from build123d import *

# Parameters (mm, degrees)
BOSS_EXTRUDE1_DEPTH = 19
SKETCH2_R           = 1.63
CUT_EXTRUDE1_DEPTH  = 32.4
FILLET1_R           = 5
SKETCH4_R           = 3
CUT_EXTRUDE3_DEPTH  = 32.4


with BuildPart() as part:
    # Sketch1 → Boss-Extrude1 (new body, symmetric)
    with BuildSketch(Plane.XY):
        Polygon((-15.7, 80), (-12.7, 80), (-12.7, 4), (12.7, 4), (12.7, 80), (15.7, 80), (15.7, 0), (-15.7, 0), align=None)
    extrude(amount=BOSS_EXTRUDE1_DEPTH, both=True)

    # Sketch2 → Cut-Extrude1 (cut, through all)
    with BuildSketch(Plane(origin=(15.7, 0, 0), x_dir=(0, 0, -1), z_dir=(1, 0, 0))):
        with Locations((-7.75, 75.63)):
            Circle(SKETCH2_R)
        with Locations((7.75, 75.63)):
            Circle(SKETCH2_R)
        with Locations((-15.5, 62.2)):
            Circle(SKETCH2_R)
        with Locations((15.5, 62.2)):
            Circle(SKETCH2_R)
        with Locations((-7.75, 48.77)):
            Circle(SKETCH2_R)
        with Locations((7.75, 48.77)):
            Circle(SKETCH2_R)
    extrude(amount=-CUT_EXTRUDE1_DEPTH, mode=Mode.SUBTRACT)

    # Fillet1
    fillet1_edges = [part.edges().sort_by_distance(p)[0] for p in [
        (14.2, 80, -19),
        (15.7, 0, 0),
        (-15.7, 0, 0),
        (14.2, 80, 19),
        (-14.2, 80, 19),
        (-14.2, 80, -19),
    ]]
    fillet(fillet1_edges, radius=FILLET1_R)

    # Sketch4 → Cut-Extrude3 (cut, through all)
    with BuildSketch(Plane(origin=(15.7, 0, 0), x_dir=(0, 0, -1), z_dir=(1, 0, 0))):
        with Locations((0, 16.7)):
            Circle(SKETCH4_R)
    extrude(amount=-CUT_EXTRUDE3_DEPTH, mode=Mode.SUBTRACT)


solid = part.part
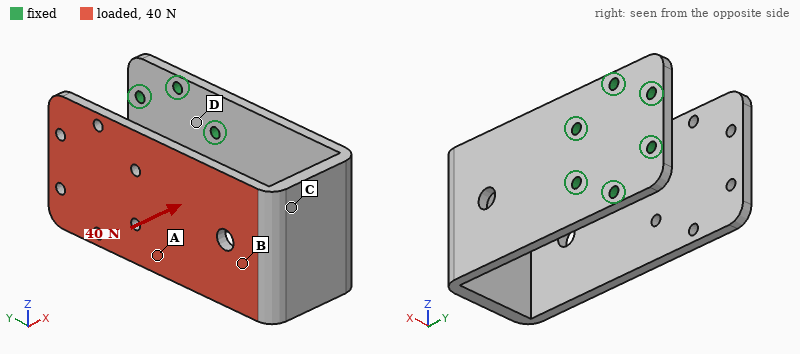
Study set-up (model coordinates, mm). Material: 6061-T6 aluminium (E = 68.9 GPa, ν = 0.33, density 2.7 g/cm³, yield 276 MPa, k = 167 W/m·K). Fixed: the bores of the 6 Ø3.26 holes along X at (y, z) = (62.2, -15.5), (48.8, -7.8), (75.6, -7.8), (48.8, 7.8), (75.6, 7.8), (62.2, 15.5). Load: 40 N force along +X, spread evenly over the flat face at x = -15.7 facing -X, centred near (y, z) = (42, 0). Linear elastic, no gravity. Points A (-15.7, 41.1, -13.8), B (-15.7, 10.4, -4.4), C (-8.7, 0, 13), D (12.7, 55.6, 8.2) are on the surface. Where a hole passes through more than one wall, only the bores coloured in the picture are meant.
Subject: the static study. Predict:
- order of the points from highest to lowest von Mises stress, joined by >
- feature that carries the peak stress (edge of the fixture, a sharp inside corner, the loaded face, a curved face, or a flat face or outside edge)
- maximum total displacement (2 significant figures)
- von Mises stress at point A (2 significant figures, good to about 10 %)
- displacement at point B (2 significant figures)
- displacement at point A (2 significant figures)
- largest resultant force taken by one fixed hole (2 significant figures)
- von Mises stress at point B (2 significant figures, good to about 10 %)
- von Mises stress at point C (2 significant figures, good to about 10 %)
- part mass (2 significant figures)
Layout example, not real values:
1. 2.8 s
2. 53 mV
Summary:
1. B > C > A > D
2. the loaded face
3. 1.0 mm
4. 7.1 MPa
5. 0.21 mm
6. 0.46 mm
7. 22 N
8. 20 MPa
9. 13 MPa
10. 57 g
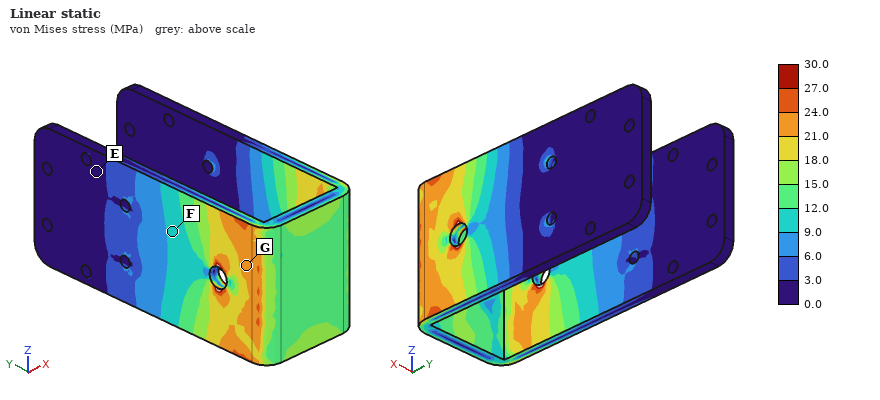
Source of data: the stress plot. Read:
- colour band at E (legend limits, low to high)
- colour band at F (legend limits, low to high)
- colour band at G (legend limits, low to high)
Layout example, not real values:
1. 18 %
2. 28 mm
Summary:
1. 0.0 to 3.0 MPa
2. 9.0 to 12.0 MPa
3. 21.0 to 24.0 MPa
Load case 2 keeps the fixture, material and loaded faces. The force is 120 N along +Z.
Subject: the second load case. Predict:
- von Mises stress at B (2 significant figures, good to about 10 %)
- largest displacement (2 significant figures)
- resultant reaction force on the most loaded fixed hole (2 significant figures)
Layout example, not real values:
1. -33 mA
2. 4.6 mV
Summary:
1. 9.5 MPa
2. 1.1 mm
3. 200 N
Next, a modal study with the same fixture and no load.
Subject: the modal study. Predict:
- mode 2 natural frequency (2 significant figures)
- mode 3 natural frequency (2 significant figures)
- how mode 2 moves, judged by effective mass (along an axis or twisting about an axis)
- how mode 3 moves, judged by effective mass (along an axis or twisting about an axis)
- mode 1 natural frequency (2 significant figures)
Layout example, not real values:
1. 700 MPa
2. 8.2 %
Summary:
1. 390 Hz
2. 430 Hz
3. along Z
4. along X
5. 220 Hz
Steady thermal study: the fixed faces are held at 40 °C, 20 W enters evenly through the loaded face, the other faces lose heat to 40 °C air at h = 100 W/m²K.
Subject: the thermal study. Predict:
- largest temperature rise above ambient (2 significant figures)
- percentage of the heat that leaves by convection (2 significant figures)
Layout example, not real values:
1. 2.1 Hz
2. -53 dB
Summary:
1. 35 K
2. 82 %
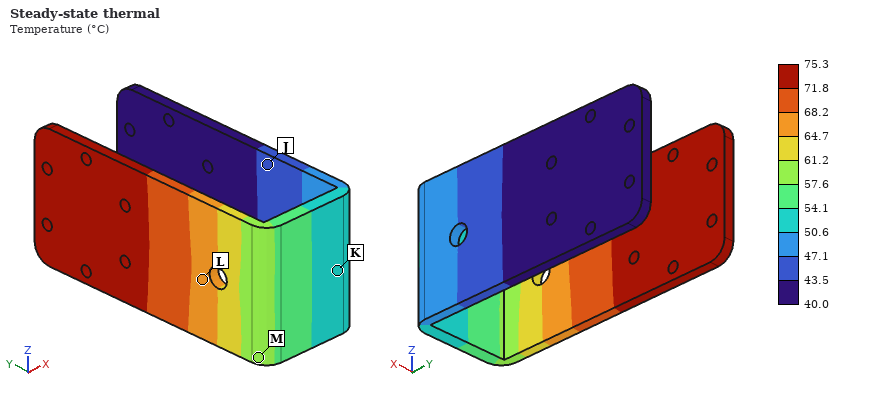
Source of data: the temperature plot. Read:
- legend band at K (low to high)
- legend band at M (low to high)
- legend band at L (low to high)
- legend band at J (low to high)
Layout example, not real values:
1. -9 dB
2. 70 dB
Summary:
1. 50.6 to 54.1 °C
2. 57.6 to 61.2 °C
3. 64.7 to 68.2 °C
4. 43.5 to 47.1 °C
